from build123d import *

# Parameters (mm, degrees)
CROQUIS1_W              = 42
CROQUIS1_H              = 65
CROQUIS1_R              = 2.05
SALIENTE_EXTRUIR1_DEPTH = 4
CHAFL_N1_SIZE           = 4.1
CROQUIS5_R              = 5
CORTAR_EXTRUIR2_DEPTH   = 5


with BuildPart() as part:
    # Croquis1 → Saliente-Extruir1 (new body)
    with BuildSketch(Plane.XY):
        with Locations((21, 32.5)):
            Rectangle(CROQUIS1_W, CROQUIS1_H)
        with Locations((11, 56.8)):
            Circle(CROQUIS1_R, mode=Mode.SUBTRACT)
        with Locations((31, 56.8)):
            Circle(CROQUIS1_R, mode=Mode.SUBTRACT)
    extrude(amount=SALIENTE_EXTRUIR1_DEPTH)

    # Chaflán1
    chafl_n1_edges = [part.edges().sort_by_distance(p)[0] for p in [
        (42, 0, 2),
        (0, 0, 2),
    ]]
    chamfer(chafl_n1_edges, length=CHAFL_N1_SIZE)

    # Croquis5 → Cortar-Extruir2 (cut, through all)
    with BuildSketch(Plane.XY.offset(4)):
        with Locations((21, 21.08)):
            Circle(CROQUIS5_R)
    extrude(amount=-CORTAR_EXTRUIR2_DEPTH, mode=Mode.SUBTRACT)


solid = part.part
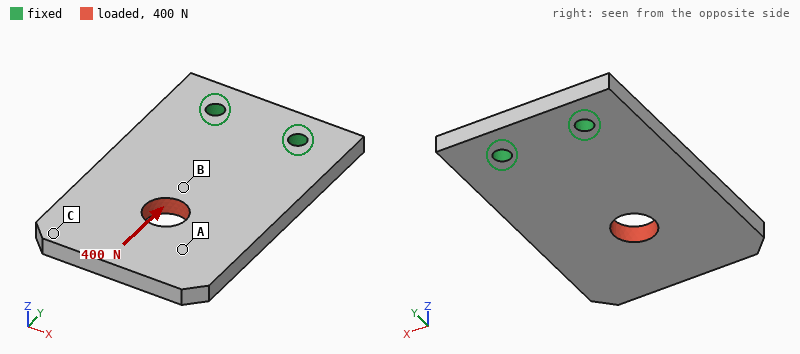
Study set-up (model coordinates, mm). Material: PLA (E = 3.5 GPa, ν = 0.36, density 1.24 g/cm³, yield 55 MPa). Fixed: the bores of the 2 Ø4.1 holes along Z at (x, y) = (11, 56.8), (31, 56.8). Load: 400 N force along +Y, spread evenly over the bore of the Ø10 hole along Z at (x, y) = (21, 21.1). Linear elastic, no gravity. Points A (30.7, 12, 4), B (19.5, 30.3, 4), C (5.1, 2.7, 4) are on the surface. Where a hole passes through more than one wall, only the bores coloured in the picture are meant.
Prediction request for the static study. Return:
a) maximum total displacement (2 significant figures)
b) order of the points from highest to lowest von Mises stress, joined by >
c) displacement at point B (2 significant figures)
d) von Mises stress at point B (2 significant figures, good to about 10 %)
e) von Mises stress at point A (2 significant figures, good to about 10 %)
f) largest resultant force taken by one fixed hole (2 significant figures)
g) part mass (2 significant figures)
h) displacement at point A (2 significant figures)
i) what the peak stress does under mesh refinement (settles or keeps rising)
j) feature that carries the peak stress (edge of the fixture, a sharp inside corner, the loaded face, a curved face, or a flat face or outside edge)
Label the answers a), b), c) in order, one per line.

a) 42 µm
b) B > A > C
c) 24 µm
d) 3.5 MPa
e) 1.6 MPa
f) 200 N
g) 13 g
h) 31 µm
i) keeps rising
j) edge of the fixture
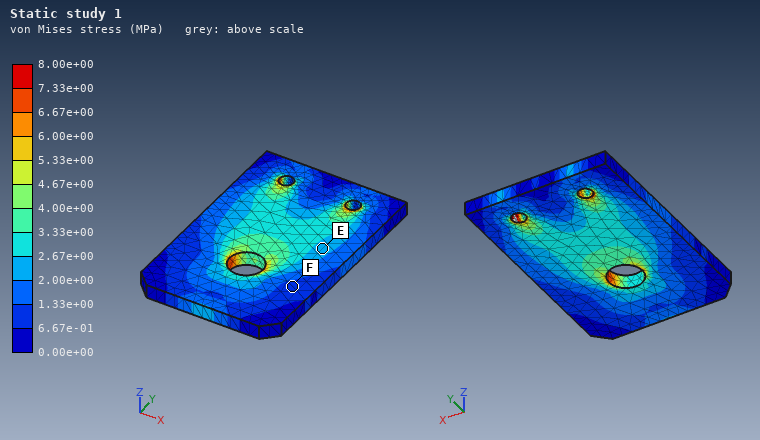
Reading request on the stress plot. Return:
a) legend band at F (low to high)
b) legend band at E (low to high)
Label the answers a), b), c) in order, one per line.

a) 6.67e-01 to 1.33e+00 MPa
b) 2.00e+00 to 2.67e+00 MPa
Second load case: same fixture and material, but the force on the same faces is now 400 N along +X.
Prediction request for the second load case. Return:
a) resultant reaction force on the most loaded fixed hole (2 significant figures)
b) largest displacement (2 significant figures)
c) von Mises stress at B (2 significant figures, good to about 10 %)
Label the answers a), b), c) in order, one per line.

a) 650 N
b) 0.35 mm
c) 7.8 MPa
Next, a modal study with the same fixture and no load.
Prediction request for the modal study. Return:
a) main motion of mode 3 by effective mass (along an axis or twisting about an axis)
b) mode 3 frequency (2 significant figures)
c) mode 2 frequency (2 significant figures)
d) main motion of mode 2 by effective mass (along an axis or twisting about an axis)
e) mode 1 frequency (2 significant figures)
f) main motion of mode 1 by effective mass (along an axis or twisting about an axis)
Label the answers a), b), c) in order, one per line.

a) along Z
b) 2000 Hz
c) 990 Hz
d) twisting about Y
e) 350 Hz
f) along Z
